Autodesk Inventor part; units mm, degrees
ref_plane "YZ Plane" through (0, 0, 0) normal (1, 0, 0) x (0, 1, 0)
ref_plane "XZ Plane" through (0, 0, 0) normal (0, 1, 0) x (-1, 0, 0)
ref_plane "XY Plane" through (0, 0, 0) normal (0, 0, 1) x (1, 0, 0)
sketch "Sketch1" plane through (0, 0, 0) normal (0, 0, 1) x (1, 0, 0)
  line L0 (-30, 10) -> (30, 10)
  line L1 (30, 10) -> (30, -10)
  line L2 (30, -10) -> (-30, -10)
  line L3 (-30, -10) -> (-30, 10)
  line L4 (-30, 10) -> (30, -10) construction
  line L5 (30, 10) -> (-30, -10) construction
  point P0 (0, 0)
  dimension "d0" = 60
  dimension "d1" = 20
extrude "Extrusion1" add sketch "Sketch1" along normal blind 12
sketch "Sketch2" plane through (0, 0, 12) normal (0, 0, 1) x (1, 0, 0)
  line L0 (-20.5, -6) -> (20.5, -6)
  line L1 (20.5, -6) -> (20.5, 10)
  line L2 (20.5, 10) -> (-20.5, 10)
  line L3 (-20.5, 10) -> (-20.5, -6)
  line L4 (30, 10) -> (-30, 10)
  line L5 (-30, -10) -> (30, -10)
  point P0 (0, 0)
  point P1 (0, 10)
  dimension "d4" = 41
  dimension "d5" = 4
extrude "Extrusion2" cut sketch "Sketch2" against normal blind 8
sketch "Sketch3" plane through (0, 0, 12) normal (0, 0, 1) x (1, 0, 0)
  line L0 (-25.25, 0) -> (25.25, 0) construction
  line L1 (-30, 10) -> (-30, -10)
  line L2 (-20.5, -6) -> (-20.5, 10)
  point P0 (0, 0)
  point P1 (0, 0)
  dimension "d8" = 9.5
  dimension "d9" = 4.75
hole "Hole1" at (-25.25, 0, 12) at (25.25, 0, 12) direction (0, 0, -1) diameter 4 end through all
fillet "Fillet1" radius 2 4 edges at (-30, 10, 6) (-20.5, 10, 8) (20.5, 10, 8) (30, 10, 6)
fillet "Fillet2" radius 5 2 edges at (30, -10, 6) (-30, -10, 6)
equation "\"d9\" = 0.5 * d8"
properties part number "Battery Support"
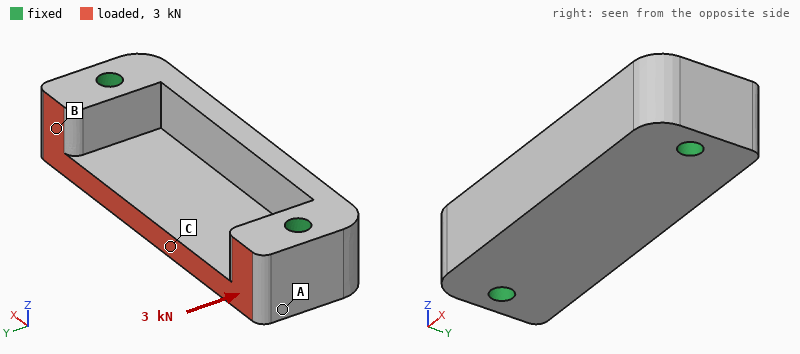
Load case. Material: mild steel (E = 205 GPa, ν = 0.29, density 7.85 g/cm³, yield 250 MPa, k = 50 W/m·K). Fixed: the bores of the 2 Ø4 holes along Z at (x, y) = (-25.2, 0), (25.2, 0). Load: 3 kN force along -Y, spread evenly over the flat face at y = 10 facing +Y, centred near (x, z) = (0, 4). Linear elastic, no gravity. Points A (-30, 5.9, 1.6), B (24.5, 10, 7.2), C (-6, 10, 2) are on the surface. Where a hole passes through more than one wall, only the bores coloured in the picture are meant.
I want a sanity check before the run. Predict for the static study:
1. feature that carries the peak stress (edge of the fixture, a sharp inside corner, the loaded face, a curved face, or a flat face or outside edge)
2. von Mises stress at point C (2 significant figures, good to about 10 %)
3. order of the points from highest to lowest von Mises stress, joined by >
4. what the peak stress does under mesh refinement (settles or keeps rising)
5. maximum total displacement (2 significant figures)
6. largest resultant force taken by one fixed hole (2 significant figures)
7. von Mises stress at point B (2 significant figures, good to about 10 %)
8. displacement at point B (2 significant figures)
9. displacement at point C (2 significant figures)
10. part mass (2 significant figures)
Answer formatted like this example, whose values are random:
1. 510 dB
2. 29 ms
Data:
1. edge of the fixture
2. 20 MPa
3. C > B > A
4. keeps rising
5. 4.4 µm
6. 1.5 kN
7. 11 MPa
8. 1.1 µm
9. 4.1 µm
10. 68 g
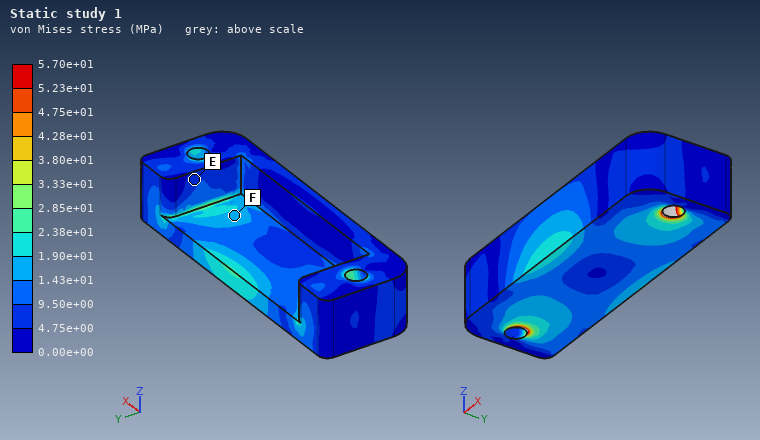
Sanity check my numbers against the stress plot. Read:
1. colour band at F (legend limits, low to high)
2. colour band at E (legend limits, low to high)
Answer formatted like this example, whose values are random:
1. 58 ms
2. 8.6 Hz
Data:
1. 1.43e+01 to 1.90e+01 MPa
2. 4.75e+00 to 9.50e+00 MPa
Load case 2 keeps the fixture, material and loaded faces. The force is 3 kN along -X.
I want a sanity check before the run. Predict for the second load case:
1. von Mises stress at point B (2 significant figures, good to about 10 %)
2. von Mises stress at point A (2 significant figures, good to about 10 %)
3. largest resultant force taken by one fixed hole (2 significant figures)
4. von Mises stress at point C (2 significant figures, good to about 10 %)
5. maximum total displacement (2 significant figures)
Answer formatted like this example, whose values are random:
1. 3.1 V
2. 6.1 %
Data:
1. 17 MPa
2. 11 MPa
3. 1.6 kN
4. 17 MPa
5. 2.1 µm
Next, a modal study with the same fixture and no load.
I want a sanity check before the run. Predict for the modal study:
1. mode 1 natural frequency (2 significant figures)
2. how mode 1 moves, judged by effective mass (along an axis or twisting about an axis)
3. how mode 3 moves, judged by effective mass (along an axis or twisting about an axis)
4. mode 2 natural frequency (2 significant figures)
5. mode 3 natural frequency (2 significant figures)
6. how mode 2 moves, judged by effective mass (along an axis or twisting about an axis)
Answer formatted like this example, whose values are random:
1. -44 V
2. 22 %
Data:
1. 12 kHz
2. along Z
3. along Y
4. 16 kHz
5. 20 kHz
6. along Y
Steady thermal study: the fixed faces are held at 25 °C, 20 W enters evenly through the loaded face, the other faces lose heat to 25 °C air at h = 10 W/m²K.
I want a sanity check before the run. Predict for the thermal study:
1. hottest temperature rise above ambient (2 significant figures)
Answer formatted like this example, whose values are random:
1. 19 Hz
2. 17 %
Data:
1. 26 K
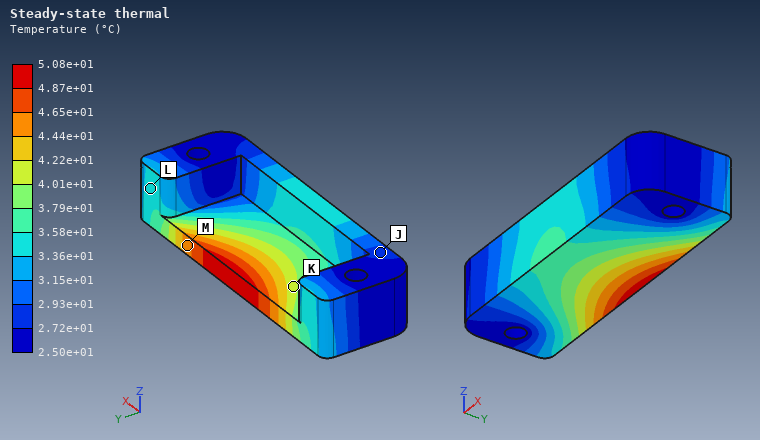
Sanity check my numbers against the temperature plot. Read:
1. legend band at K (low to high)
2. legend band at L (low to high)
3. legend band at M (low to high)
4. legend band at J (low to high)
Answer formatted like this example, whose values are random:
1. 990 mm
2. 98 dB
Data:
1. 4.01e+01 to 4.22e+01 °C
2. 3.36e+01 to 3.58e+01 °C
3. 4.44e+01 to 4.65e+01 °C
4. 2.72e+01 to 2.93e+01 °C
